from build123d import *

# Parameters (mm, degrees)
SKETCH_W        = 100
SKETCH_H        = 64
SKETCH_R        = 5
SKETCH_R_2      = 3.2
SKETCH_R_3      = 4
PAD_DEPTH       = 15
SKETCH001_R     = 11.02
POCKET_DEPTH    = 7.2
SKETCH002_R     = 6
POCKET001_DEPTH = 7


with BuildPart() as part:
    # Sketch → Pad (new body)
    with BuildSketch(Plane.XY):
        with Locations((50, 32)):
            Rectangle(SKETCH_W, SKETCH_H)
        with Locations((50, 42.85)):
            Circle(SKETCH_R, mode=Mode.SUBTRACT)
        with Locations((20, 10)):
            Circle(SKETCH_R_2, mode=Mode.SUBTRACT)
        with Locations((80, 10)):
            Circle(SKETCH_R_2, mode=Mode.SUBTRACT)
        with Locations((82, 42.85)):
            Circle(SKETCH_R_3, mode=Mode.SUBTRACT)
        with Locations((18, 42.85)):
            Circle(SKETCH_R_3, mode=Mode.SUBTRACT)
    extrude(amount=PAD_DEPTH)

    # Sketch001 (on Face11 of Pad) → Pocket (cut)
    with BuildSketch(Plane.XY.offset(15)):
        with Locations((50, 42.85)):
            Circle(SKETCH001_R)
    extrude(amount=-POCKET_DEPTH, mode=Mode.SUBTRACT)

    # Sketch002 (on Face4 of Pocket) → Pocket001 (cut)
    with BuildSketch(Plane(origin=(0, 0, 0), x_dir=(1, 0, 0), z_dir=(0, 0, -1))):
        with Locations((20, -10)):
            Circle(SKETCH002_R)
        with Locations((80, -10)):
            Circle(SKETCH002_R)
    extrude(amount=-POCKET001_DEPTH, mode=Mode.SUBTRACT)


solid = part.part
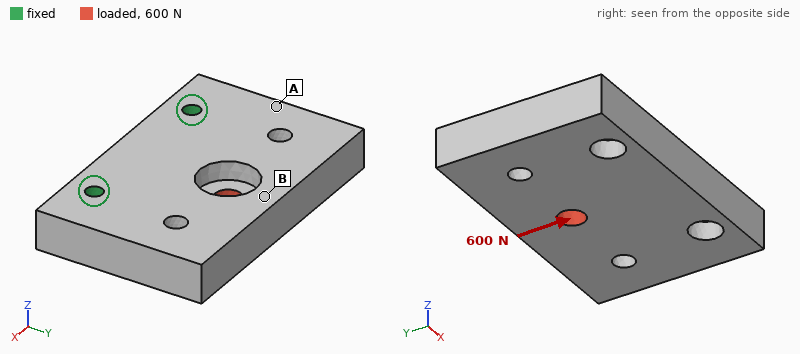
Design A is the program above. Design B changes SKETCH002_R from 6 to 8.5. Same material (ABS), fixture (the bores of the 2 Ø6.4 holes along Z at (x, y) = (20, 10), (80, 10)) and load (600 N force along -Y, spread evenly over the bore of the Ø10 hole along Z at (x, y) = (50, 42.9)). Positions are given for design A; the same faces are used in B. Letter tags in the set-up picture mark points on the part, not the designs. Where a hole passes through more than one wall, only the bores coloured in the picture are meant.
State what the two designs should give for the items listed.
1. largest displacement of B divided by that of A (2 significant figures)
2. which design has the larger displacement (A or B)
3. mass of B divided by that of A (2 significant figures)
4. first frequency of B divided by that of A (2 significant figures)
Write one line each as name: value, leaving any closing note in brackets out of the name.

largest displacement of B divided by that of A: 1.1
which design has the larger displacement: B
mass of B divided by that of A: 0.98
first frequency of B divided by that of A: 0.96
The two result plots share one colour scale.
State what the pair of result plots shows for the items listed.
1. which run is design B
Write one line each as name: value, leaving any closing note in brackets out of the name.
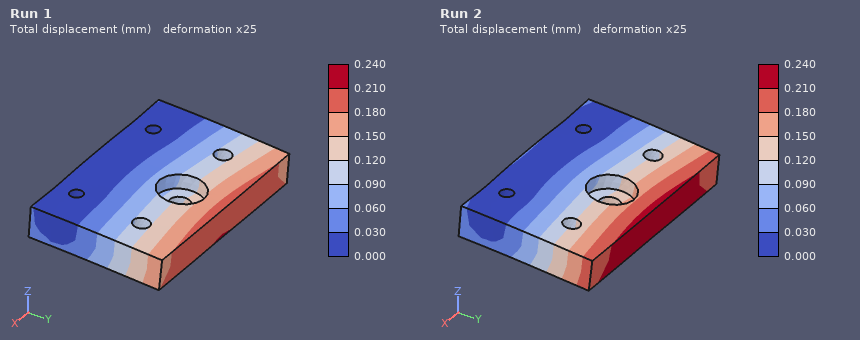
which run is design B: Run 2
